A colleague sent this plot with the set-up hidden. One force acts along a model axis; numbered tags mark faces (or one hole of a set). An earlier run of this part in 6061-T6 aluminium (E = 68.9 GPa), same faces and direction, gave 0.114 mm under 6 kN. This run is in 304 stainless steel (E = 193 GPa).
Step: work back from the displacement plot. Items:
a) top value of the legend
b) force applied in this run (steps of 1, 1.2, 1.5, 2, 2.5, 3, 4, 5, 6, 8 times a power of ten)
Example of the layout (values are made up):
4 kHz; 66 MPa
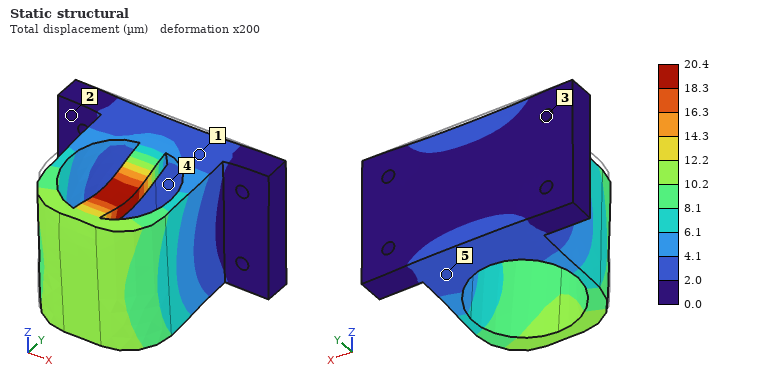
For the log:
20.4 µm; 3 kN
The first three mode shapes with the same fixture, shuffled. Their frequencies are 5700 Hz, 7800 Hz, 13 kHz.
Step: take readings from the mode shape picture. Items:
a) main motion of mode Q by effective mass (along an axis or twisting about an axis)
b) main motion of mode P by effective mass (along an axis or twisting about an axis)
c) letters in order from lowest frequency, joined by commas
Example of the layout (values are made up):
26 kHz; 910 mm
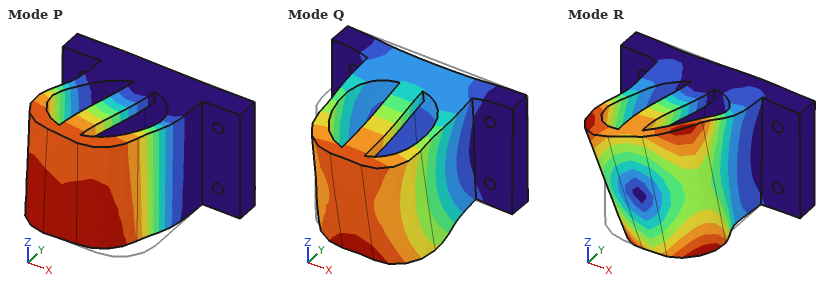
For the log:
along Z; along X; P, Q, R
